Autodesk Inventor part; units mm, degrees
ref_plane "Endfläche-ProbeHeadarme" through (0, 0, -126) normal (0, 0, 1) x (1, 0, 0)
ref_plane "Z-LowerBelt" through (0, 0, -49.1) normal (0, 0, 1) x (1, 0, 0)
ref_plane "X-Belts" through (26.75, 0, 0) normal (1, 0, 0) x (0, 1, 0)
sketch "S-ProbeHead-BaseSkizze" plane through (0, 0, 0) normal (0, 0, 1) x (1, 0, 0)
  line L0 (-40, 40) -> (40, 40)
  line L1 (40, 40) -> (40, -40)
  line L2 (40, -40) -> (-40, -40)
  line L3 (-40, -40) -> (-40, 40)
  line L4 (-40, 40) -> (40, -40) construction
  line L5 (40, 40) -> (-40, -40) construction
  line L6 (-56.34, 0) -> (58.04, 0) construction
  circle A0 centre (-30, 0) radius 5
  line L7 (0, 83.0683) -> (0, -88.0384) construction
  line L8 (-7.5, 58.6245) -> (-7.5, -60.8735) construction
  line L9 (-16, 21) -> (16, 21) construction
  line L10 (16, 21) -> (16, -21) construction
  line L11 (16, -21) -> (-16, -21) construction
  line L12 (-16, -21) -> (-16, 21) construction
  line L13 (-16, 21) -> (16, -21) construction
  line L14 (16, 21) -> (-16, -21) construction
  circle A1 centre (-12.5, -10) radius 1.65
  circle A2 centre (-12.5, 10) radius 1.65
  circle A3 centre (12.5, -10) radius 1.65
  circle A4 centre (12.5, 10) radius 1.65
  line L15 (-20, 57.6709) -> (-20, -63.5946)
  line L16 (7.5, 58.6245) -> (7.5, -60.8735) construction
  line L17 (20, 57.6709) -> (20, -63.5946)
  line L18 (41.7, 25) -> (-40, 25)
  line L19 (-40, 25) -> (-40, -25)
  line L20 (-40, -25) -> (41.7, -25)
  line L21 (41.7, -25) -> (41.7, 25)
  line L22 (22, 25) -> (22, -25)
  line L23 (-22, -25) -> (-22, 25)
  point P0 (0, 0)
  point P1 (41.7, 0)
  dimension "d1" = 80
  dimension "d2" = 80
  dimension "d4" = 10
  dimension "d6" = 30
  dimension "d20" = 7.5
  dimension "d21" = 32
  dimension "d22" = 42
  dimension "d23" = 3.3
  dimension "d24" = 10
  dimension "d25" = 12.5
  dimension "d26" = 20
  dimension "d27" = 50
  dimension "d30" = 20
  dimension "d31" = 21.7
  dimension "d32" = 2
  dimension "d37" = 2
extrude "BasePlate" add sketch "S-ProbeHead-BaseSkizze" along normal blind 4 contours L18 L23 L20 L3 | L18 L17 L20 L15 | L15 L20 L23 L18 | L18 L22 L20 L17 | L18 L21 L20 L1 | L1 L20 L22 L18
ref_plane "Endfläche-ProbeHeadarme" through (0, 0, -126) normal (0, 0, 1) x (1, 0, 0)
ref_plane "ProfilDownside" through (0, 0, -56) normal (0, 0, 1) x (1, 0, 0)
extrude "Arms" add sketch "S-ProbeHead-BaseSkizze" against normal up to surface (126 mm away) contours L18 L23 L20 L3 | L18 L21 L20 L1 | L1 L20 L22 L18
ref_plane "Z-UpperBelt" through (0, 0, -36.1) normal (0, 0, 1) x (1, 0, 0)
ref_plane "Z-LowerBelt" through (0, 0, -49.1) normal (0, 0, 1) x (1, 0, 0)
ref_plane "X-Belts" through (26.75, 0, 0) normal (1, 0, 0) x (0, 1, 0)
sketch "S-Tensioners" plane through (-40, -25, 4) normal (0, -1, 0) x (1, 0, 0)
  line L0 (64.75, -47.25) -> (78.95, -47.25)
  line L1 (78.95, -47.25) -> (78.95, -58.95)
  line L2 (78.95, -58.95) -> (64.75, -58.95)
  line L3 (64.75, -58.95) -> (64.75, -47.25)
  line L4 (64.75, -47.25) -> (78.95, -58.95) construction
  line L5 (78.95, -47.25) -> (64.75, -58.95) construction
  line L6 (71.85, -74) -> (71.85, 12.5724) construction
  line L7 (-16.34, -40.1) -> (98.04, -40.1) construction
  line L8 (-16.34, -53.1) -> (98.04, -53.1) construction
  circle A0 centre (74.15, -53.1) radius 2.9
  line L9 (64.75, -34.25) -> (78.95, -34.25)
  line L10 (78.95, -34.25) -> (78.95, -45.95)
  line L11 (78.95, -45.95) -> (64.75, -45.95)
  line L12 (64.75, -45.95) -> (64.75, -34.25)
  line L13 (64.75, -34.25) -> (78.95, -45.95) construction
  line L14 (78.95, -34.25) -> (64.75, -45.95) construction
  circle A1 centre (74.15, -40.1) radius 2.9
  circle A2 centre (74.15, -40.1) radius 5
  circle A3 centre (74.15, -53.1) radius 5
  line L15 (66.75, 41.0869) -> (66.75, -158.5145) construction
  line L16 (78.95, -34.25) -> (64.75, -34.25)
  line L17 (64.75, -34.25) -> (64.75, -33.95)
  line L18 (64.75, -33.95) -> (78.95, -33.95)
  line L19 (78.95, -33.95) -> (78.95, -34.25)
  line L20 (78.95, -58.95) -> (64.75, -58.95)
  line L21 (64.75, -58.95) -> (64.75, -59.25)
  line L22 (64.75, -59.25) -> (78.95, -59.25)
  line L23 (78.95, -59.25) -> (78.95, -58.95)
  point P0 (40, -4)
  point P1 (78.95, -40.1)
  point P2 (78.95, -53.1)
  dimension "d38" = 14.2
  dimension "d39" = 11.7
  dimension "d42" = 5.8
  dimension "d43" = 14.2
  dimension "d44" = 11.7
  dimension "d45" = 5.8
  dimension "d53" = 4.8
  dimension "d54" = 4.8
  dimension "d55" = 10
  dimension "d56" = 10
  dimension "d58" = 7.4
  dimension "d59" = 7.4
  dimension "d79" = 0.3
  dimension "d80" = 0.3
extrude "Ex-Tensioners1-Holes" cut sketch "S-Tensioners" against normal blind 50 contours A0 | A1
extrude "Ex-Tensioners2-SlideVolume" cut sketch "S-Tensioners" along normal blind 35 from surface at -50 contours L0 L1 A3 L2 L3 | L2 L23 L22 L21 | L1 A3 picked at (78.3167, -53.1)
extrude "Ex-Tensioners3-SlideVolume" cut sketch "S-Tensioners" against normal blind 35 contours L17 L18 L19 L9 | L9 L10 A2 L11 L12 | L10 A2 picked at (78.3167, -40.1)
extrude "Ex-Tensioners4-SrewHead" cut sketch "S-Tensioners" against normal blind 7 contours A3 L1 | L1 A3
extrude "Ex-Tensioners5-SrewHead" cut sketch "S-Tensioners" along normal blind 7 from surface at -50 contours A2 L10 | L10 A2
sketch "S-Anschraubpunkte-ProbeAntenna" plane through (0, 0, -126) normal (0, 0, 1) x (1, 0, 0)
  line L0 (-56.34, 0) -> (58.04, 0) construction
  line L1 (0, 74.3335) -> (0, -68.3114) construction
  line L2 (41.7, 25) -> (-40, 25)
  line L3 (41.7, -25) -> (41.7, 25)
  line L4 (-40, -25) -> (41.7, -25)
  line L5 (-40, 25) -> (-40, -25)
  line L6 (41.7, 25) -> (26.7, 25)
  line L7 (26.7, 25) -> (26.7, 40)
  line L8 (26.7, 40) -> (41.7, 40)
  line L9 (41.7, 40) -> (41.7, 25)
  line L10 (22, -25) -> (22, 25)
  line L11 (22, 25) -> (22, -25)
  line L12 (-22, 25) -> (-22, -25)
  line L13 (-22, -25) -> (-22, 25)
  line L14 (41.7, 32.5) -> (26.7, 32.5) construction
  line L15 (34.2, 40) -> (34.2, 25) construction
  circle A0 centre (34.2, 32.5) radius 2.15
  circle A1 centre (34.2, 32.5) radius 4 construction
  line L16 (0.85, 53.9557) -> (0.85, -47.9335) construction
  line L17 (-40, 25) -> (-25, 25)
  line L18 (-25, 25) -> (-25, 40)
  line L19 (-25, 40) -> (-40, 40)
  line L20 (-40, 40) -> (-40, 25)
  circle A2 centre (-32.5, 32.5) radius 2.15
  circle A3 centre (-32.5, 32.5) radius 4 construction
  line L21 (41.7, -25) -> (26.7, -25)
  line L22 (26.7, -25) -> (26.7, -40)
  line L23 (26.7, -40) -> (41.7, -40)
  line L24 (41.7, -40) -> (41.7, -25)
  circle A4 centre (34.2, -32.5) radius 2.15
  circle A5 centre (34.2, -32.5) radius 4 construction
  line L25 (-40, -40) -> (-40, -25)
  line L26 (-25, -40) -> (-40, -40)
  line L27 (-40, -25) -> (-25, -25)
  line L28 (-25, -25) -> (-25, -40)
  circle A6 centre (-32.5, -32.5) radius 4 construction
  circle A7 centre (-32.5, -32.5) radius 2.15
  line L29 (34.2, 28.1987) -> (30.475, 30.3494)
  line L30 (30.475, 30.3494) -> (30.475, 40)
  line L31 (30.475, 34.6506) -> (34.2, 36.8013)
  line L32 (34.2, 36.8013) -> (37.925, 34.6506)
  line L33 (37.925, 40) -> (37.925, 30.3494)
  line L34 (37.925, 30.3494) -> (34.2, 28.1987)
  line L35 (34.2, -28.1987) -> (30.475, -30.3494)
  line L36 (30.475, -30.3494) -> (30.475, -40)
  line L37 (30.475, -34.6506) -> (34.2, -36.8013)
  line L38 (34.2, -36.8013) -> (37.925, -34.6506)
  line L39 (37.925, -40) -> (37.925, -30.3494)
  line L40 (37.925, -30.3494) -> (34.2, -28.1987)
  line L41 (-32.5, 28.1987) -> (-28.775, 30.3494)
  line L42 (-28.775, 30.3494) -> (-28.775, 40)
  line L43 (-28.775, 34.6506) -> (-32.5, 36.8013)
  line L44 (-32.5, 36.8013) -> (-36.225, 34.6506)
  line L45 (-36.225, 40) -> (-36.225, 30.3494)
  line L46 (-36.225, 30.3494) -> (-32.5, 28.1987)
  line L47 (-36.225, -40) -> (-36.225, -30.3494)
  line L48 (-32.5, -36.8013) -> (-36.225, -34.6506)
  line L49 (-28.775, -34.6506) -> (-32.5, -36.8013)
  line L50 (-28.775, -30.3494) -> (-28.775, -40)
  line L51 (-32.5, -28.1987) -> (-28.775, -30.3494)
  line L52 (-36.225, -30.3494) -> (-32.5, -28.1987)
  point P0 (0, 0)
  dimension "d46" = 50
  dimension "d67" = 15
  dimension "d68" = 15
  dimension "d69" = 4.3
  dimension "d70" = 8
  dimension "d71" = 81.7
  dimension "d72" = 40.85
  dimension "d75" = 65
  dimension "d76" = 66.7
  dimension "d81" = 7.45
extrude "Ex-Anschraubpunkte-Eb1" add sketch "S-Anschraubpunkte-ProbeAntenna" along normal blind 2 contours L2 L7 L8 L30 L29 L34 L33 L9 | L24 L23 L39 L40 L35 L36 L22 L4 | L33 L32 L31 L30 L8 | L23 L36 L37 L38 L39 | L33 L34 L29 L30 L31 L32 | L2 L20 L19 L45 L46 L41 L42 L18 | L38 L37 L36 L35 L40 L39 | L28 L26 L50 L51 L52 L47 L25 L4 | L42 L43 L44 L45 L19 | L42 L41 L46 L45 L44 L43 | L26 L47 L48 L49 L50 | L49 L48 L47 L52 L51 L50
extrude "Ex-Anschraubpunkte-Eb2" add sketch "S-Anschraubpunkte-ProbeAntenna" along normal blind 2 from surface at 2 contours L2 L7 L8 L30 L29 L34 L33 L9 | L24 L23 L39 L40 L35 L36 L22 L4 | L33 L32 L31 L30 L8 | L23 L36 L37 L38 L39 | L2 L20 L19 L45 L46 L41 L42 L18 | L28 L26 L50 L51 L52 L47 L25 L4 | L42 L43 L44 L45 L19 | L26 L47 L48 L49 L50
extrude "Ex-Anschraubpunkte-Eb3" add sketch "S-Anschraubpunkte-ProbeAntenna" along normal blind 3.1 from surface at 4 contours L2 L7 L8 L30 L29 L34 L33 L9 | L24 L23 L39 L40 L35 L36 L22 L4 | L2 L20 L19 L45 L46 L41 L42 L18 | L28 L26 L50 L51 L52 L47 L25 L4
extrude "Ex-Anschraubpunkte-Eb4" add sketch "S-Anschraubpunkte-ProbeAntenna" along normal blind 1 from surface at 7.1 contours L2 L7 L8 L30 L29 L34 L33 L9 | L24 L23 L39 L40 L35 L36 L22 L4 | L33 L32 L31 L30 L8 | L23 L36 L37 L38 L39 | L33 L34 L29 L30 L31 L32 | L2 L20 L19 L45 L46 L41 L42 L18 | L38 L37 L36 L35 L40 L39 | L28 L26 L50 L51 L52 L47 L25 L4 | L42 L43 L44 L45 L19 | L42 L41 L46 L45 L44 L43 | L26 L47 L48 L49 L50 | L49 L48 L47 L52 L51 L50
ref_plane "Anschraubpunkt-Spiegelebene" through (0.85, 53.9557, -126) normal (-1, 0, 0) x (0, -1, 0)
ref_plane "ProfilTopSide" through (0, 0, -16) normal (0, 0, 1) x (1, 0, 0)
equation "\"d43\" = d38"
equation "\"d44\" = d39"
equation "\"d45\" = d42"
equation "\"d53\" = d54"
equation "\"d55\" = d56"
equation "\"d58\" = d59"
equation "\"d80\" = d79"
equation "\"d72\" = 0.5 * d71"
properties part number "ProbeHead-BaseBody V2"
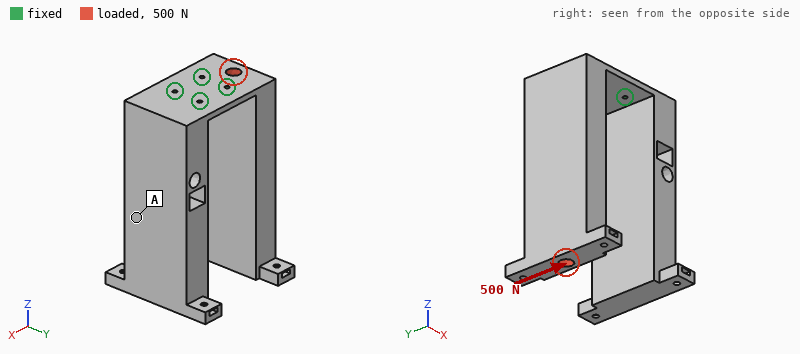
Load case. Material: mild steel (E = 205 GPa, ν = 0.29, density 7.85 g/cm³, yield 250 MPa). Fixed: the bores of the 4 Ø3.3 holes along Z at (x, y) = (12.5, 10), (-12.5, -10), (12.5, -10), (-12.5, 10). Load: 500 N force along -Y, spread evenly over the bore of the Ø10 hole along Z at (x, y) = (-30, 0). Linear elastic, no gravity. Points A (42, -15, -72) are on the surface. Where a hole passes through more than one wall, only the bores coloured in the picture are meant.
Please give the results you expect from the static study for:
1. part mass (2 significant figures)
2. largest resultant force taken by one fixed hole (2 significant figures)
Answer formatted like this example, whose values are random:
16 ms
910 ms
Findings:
1.9 kg
1.3 kN
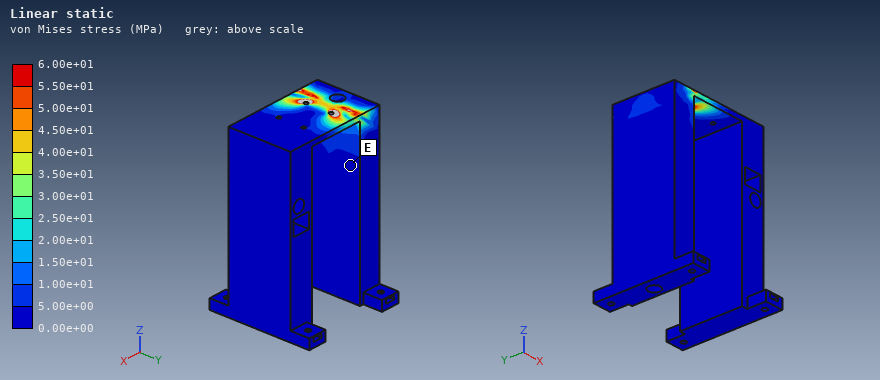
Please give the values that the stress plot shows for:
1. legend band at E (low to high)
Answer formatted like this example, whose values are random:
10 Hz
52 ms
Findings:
0.00e+00 to 5.00e+00 MPa
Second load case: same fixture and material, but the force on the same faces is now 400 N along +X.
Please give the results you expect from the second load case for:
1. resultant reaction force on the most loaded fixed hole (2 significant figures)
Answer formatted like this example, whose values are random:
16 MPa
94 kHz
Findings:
250 N
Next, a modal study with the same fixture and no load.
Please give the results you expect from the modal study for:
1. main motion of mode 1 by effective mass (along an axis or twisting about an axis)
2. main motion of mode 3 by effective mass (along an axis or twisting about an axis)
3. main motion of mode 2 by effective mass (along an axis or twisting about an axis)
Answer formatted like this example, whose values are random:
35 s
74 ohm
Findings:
along X
along Y
along X
